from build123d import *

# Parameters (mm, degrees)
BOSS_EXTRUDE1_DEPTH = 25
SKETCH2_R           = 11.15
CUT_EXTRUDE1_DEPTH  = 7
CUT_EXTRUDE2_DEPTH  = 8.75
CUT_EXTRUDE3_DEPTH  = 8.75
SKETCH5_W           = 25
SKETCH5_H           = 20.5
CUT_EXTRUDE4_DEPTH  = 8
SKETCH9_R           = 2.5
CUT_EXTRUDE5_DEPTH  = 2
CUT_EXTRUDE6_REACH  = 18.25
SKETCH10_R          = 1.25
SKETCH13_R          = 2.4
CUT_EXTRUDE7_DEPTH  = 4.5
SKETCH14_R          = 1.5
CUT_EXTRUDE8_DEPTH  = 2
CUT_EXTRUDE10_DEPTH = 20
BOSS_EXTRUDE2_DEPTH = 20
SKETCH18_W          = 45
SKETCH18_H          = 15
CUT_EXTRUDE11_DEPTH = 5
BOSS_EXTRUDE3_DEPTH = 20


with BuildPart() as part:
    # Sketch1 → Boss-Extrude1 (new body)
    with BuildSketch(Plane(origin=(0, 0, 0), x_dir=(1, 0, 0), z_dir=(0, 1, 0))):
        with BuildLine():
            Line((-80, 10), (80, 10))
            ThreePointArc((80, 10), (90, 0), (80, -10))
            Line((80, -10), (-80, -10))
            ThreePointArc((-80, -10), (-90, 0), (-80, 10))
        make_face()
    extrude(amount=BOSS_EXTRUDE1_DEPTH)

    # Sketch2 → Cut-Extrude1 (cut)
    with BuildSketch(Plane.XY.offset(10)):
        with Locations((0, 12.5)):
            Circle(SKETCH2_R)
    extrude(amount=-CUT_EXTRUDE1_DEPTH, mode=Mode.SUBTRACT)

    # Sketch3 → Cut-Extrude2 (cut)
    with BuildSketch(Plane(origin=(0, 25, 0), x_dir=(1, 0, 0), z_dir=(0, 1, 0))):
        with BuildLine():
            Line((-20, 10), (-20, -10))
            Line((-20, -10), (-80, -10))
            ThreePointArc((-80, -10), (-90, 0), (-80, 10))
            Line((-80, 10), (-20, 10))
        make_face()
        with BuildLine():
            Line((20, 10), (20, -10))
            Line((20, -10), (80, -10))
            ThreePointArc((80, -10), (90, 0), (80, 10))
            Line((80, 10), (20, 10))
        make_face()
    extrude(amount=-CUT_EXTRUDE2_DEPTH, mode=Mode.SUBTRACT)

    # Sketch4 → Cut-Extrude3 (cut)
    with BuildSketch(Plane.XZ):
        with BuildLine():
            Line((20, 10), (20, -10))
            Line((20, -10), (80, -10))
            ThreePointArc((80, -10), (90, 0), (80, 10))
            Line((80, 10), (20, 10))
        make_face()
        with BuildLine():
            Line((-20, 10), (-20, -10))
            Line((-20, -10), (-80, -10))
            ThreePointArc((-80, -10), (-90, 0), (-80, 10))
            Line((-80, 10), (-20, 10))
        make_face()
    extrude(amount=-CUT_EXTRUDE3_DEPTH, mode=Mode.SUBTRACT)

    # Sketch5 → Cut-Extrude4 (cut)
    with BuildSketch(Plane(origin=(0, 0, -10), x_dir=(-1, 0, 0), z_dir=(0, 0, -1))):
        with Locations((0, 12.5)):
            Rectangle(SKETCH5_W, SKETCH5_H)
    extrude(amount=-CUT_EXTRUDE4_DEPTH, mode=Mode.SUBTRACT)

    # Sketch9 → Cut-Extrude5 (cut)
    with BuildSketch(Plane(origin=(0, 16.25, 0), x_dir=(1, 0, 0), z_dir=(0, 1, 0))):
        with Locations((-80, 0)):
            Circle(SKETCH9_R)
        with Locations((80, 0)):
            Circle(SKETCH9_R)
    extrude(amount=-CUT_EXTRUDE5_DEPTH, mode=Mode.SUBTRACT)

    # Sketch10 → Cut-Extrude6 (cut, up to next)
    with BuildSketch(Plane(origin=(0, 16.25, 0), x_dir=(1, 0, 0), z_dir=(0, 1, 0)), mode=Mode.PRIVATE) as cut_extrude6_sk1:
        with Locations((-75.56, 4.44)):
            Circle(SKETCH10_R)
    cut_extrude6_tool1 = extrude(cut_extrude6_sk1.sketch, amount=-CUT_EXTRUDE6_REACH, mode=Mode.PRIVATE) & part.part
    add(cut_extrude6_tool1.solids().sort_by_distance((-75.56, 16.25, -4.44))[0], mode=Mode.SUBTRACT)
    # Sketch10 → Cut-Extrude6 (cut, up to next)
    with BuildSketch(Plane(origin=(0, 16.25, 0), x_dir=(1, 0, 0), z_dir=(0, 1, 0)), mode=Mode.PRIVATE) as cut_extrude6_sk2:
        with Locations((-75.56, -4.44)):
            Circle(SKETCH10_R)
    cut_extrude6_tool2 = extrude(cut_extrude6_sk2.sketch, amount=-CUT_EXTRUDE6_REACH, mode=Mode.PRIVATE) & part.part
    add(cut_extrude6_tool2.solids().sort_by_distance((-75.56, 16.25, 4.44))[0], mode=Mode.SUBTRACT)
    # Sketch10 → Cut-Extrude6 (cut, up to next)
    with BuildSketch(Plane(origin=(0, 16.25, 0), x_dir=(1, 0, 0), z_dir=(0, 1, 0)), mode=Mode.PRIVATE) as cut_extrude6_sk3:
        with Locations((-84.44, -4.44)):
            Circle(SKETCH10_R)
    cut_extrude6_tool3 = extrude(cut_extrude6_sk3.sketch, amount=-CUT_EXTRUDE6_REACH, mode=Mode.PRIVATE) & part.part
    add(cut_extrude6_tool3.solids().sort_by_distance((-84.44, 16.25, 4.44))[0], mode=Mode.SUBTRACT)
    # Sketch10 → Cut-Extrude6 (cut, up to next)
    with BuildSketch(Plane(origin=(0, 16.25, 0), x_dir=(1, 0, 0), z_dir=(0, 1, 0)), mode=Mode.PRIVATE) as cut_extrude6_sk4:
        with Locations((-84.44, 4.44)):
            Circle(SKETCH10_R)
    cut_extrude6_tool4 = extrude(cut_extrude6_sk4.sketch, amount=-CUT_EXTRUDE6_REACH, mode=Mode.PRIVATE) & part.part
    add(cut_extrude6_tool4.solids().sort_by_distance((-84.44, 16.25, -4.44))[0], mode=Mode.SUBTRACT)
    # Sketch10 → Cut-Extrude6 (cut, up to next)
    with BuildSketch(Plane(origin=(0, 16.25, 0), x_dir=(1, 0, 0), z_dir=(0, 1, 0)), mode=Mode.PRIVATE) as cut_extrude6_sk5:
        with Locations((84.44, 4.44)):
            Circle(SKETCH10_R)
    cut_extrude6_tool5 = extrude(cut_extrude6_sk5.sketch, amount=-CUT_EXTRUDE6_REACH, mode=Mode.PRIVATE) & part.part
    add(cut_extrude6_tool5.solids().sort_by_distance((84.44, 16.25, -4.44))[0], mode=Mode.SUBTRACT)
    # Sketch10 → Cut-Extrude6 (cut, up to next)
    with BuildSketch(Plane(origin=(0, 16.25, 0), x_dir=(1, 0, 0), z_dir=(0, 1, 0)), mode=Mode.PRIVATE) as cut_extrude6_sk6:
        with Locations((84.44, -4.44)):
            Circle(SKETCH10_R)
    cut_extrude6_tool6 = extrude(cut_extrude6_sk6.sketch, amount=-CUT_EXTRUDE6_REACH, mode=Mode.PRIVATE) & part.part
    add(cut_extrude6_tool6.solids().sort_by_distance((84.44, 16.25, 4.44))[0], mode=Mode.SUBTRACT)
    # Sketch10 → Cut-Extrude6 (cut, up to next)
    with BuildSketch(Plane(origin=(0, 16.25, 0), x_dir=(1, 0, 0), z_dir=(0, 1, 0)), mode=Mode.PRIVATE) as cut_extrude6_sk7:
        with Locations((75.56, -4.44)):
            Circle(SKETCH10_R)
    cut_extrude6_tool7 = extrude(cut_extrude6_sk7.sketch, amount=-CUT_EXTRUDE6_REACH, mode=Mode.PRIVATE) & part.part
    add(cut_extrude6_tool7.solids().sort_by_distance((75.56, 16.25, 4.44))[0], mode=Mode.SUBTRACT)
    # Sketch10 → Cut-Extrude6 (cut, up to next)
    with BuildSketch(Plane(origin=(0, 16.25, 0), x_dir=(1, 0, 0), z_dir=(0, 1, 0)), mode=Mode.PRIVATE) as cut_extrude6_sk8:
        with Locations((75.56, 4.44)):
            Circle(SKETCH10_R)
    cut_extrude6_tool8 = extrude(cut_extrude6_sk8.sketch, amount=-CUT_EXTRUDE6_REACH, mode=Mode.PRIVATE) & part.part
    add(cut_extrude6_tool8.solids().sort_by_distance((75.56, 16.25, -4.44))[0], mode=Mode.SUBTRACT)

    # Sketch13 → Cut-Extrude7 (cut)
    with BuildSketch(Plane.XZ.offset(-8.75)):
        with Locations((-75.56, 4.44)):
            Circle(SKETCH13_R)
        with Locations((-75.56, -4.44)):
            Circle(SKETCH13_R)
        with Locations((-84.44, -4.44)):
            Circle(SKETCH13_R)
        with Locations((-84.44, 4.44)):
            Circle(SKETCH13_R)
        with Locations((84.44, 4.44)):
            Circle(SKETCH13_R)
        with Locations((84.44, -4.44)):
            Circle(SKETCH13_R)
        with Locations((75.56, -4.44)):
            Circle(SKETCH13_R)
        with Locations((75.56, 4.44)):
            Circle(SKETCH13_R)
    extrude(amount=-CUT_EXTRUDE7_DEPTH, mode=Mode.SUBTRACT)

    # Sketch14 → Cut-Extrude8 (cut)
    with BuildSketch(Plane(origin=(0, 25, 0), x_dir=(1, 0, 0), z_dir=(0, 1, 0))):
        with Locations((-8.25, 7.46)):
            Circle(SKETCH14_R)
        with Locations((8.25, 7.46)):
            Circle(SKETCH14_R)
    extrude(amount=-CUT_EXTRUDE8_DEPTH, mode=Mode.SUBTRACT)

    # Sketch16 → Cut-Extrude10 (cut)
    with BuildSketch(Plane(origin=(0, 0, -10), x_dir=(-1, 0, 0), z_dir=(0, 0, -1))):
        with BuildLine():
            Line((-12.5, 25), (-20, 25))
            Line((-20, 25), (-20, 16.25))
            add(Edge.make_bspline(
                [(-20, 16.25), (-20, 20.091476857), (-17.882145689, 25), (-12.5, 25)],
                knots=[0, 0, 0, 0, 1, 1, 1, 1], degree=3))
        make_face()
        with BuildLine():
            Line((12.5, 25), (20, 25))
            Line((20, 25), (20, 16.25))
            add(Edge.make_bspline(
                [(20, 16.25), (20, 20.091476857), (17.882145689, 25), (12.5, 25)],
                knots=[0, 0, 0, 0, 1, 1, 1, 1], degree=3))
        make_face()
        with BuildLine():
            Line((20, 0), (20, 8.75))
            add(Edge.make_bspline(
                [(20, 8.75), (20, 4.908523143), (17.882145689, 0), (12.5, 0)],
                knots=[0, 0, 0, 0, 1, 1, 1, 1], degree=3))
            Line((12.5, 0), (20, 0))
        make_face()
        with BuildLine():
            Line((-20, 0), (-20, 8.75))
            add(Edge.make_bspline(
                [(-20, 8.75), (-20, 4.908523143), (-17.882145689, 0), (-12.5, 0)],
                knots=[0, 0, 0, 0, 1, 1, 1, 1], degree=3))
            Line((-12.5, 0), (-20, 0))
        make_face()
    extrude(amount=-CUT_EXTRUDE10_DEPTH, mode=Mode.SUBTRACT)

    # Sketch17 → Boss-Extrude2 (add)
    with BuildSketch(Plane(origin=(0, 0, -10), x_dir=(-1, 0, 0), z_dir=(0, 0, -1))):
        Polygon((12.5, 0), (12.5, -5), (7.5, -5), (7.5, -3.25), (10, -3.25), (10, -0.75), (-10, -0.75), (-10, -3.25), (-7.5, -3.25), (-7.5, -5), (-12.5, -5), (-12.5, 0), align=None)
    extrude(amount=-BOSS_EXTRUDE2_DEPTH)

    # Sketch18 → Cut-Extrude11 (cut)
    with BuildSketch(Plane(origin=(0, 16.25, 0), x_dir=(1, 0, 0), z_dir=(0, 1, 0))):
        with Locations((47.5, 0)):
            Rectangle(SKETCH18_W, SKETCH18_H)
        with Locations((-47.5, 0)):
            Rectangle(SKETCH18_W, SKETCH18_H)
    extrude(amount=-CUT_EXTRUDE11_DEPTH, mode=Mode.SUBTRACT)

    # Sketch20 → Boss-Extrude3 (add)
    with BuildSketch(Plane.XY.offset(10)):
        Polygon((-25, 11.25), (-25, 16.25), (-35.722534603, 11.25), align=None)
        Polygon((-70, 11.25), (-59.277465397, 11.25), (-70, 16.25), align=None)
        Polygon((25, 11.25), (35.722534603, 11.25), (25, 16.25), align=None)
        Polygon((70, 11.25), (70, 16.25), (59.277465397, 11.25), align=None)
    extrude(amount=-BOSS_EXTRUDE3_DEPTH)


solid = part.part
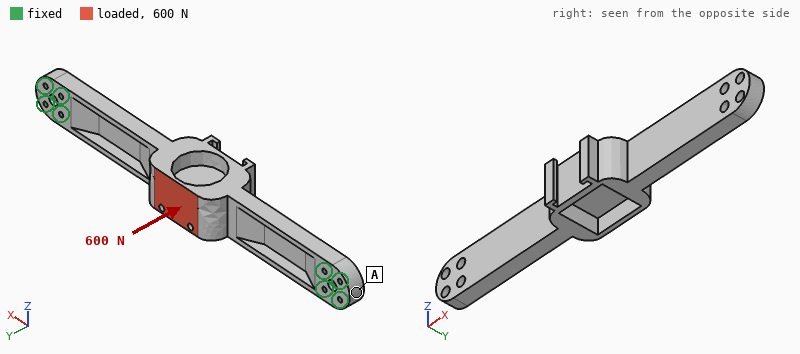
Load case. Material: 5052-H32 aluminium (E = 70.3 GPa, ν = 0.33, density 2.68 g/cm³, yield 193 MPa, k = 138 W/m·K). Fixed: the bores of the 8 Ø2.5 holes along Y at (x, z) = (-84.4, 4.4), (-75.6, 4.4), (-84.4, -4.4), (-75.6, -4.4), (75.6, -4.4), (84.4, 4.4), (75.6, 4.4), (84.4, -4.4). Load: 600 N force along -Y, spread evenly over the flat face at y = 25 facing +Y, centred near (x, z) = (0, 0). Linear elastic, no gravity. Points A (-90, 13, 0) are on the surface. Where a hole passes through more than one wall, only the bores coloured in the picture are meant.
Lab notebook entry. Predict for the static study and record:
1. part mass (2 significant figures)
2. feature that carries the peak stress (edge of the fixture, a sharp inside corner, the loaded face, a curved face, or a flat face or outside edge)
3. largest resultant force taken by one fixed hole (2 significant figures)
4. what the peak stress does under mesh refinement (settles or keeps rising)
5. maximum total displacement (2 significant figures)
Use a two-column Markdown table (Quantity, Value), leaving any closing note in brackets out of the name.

| Quantity | Value |
|---|---|
| part mass | 74 g |
| feature that carries the peak stress | edge of the fixture |
| largest resultant force taken by one fixed hole | 560 N |
| what the peak stress does under mesh refinement | keeps rising |
| maximum total displacement | 0.19 mm |
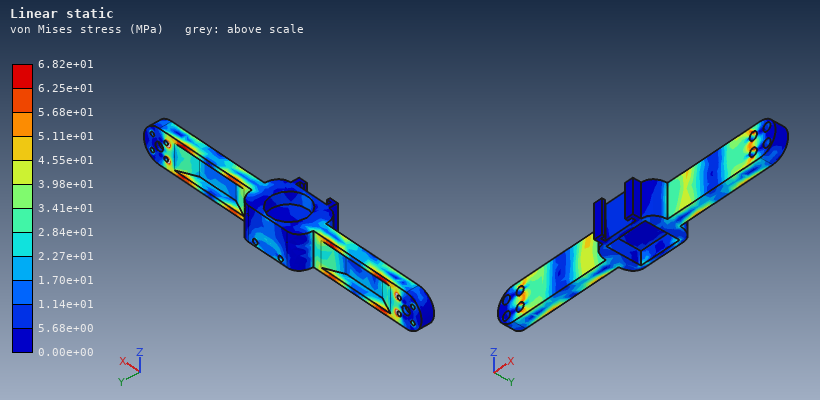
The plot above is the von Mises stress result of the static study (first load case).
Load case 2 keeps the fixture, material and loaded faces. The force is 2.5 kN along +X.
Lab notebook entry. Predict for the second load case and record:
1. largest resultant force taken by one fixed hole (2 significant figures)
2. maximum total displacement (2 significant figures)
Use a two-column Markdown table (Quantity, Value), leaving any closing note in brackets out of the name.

| Quantity | Value |
|---|---|
| largest resultant force taken by one fixed hole | 620 N |
| maximum total displacement | 0.11 mm |
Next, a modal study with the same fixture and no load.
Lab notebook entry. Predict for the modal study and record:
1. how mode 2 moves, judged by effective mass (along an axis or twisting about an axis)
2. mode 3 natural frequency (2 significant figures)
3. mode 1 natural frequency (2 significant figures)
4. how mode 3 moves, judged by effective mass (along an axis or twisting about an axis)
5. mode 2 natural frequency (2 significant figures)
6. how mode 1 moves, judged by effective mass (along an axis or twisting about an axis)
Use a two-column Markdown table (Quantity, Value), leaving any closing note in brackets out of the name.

| Quantity | Value |
|---|---|
| how mode 2 moves, judged by effective mass | along Z |
| mode 3 natural frequency | 2600 Hz |
| mode 1 natural frequency | 1300 Hz |
| how mode 3 moves, judged by effective mass | along Z |
| mode 2 natural frequency | 1600 Hz |
| how mode 1 moves, judged by effective mass | along Y |
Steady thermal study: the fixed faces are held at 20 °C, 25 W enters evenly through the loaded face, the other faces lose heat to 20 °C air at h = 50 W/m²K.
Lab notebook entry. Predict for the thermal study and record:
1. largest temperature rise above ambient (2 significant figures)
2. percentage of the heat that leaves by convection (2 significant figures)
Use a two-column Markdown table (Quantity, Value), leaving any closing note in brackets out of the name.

| Quantity | Value |
|---|---|
| largest temperature rise above ambient | 42 K |
| percentage of the heat that leaves by convection | 54 % |
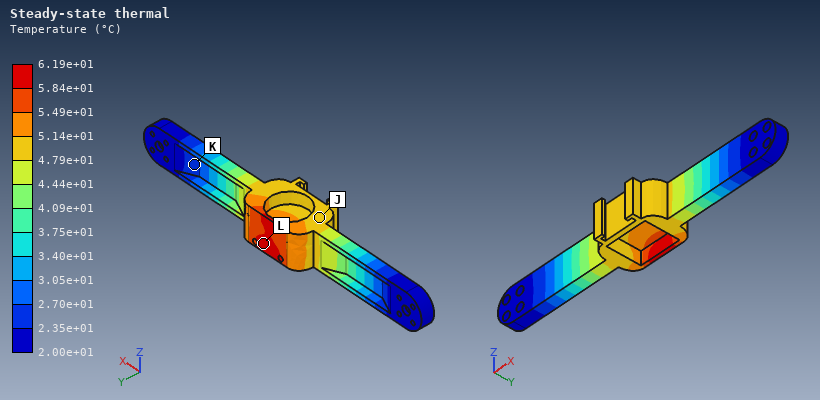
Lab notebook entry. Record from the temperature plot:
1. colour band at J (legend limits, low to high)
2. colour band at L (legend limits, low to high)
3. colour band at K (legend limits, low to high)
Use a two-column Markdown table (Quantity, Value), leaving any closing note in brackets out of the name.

| Quantity | Value |
|---|---|
| colour band at J | 4.79e+01 to 5.14e+01 °C |
| colour band at L | 5.84e+01 to 6.19e+01 °C |
| colour band at K | 2.35e+01 to 2.70e+01 °C |
